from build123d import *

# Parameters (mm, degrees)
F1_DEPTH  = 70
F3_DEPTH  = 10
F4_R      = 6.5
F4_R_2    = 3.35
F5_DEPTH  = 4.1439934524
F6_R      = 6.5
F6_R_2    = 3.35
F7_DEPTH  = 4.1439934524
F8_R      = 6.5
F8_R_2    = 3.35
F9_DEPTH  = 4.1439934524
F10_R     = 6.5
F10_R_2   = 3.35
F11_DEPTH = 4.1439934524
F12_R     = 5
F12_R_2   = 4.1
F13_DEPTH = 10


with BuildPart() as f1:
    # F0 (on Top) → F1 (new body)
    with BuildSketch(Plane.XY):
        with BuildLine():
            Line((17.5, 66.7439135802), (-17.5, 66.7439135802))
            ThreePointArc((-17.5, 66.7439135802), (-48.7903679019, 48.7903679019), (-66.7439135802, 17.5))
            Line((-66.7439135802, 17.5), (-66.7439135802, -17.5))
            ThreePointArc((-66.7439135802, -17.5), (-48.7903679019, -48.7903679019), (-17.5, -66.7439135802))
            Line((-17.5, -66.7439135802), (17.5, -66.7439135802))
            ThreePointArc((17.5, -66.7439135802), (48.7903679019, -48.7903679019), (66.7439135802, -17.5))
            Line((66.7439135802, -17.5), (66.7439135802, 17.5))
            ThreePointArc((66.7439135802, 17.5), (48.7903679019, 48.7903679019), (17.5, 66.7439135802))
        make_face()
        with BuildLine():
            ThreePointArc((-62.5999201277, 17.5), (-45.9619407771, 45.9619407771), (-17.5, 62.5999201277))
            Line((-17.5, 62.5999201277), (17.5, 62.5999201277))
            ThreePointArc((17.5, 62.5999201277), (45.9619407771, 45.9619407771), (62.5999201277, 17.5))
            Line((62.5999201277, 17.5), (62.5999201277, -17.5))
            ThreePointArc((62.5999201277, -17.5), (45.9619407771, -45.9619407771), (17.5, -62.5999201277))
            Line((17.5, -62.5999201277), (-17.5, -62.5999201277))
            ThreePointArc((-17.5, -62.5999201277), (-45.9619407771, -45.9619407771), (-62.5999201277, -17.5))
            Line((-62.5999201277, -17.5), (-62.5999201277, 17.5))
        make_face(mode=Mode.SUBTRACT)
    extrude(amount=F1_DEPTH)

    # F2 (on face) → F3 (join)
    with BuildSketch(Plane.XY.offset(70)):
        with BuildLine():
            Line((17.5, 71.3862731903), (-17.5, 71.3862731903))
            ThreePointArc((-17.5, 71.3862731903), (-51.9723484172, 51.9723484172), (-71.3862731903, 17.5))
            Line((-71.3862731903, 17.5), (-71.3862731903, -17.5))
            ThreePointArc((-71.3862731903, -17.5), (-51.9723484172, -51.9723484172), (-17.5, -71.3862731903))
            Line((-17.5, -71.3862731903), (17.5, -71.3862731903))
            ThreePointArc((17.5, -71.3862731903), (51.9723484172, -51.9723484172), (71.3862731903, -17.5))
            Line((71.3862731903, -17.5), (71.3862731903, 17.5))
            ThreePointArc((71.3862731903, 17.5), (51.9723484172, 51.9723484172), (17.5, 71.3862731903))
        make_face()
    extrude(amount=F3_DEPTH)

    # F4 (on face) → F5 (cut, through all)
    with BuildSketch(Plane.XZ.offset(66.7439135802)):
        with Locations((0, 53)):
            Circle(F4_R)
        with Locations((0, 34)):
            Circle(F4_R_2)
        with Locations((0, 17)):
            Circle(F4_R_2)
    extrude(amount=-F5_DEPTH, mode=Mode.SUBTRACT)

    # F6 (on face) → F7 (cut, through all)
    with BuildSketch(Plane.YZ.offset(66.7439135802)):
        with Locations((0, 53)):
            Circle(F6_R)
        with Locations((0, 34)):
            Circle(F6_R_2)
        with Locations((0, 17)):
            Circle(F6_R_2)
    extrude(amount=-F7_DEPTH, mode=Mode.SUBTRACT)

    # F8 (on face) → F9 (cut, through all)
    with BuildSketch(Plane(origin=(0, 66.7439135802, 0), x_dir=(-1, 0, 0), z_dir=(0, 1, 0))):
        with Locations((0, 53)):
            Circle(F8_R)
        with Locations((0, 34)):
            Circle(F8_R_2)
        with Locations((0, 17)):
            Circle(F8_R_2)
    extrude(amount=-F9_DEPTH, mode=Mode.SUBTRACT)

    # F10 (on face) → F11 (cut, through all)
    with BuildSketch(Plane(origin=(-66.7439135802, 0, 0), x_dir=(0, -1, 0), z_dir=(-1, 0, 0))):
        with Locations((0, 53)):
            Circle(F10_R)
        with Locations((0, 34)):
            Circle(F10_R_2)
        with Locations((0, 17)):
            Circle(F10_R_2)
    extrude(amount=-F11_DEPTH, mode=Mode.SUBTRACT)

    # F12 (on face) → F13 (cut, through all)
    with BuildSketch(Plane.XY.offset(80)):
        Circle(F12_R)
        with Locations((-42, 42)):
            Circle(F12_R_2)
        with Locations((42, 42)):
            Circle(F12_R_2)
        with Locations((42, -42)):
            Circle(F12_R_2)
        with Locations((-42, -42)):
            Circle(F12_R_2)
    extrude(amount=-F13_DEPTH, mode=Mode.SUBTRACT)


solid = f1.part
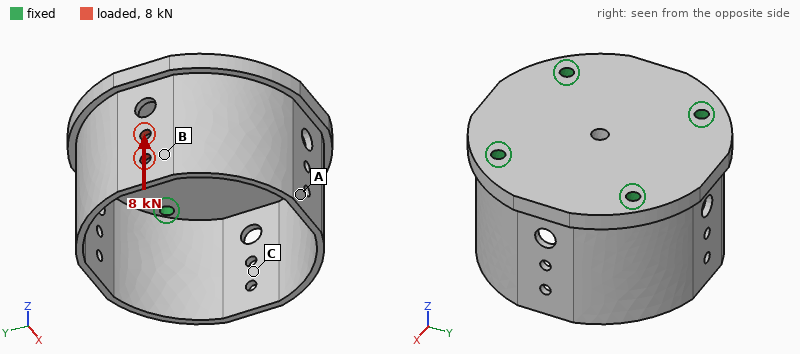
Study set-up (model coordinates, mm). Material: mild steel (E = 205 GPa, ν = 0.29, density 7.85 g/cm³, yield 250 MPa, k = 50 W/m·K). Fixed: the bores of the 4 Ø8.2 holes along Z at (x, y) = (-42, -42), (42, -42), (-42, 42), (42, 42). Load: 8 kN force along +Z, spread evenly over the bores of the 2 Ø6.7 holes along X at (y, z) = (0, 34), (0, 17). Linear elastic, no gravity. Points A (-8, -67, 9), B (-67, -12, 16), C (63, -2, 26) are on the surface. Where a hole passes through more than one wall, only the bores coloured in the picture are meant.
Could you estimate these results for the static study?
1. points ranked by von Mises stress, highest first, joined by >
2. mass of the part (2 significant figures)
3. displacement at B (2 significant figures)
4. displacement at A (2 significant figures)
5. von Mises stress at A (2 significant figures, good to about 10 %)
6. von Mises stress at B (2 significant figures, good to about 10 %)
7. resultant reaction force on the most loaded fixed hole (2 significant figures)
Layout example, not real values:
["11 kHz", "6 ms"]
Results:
["B > A > C", "2.2 kg", "0.076 mm", "0.049 mm", "15 MPa", "42 MPa", "4.6 kN"]
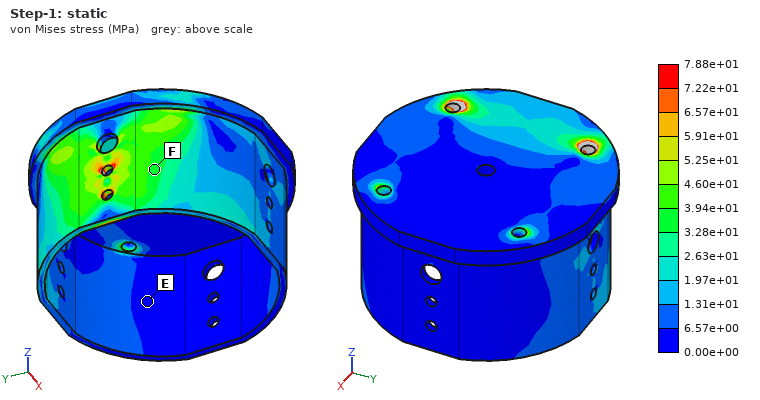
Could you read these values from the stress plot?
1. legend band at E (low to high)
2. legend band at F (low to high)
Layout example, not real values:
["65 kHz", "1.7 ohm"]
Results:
["0.00e+00 to 6.57e+00 MPa", "3.28e+01 to 3.94e+01 MPa"]
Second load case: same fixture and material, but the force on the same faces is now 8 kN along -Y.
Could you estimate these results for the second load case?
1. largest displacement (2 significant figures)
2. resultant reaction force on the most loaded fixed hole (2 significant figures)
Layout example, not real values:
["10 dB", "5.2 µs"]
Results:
["78 µm", "6.7 kN"]
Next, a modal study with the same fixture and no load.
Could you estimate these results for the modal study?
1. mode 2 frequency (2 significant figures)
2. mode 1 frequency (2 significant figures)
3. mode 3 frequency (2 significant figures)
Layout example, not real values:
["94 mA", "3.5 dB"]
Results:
["2300 Hz", "1700 Hz", "2300 Hz"]
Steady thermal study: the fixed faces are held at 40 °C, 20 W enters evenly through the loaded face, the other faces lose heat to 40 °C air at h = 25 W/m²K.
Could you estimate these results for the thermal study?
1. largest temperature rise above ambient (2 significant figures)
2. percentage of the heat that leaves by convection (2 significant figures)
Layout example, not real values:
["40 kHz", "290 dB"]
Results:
["46 K", "51 %"]
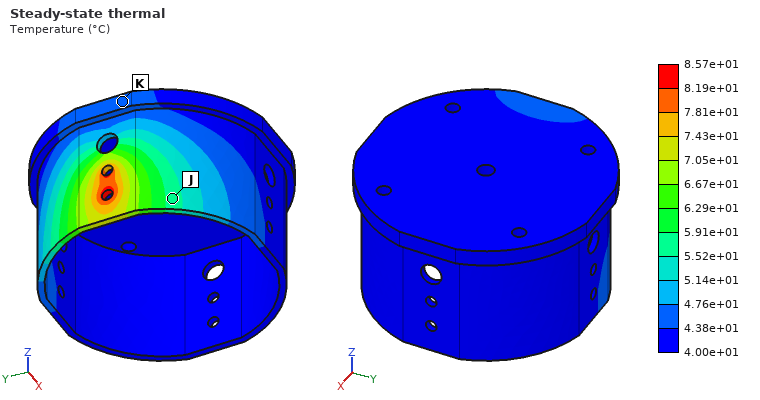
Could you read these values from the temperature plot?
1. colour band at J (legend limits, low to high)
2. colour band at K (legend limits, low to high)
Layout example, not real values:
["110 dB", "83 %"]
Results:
["5.52e+01 to 5.91e+01 °C", "4.38e+01 to 4.76e+01 °C"]
